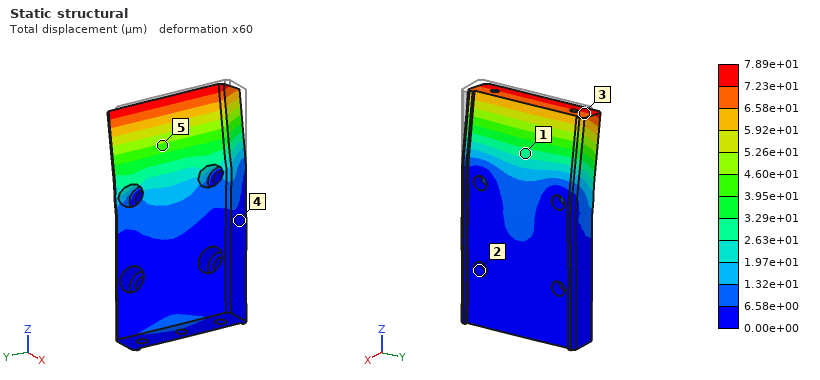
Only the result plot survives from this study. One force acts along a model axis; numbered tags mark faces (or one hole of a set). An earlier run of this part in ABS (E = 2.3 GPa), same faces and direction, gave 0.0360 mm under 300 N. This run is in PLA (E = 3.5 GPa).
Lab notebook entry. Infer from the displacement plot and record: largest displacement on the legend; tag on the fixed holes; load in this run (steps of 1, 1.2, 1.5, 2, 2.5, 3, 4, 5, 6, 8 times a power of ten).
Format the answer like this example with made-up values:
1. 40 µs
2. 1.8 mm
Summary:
1. 7.89e+01 µm
2. 2
3. 1 kN
